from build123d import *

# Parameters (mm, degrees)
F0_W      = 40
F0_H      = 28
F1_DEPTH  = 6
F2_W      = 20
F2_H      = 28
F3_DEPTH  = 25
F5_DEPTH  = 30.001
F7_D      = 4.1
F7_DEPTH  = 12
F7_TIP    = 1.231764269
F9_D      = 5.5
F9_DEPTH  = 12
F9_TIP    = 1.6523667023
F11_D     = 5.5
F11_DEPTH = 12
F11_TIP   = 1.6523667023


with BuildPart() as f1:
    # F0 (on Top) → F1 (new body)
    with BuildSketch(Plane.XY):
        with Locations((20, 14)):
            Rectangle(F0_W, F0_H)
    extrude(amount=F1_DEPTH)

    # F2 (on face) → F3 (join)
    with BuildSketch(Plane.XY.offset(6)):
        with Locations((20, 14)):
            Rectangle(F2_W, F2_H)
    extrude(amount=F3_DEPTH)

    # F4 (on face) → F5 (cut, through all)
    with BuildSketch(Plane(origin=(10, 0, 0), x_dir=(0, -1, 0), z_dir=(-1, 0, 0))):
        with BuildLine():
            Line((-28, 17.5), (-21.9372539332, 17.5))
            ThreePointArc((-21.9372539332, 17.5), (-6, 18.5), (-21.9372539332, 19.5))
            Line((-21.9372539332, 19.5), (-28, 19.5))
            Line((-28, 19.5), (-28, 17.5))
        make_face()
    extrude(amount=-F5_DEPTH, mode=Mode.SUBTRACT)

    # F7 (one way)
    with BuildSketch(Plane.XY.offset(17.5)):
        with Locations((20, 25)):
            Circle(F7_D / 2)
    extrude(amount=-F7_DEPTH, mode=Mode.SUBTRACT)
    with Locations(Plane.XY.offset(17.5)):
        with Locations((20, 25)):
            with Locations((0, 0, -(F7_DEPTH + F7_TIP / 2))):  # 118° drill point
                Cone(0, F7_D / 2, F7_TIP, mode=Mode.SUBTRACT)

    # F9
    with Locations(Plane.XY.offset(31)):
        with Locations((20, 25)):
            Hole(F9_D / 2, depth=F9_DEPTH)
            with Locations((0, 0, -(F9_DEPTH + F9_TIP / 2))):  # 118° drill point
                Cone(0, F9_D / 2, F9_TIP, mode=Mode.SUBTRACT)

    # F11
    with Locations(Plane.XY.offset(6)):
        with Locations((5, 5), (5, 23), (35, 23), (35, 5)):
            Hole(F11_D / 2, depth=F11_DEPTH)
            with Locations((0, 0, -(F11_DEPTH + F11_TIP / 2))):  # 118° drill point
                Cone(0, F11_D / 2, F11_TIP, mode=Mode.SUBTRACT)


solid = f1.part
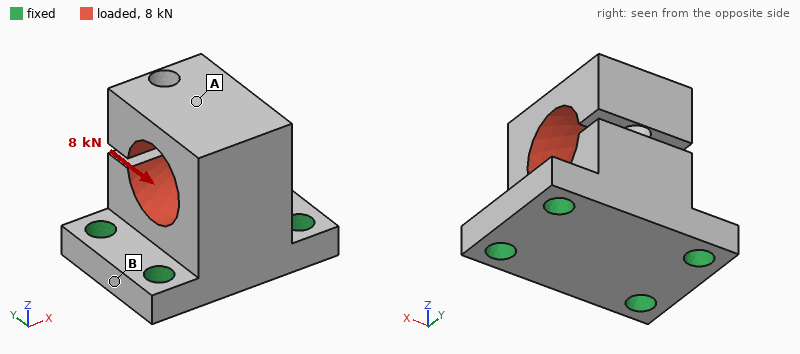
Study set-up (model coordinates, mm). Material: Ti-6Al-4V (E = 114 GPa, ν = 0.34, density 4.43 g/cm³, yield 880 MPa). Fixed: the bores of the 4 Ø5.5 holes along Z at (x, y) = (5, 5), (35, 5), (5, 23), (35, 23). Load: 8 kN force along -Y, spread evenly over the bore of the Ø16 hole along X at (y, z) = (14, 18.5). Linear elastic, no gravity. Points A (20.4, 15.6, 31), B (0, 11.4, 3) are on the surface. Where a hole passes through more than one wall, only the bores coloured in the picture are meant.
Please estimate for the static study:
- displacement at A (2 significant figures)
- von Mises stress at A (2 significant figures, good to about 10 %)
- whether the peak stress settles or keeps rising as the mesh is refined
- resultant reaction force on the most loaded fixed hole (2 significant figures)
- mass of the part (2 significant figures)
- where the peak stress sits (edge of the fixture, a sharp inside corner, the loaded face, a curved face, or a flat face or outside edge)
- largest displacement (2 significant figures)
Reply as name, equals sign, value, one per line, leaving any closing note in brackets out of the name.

displacement at A = 0.19 mm
von Mises stress at A = 79 MPa
whether the peak stress settles or keeps rising as the mesh is refined = keeps rising
resultant reaction force on the most loaded fixed hole = 4.2 kN
mass of the part = 68 g
where the peak stress sits = edge of the fixture
largest displacement = 0.22 mm
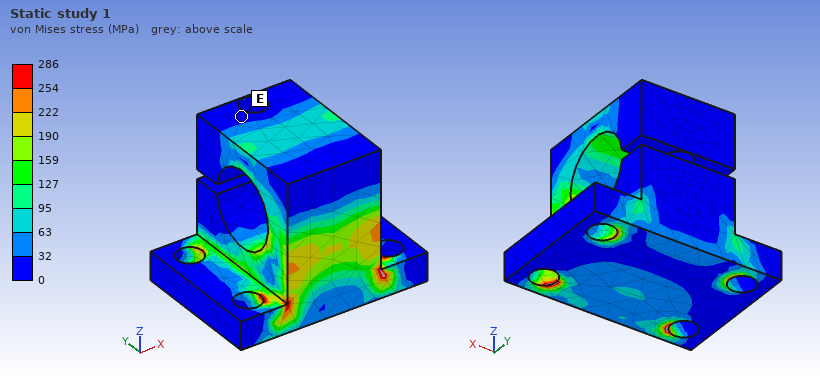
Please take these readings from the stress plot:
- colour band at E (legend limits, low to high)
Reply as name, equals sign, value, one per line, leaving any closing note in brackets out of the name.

colour band at E = 0 to 32 MPa
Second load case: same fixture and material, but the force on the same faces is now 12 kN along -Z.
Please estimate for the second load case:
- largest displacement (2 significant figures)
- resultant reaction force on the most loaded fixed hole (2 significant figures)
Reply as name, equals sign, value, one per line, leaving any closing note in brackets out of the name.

largest displacement = 0.66 mm
resultant reaction force on the most loaded fixed hole = 3.4 kN
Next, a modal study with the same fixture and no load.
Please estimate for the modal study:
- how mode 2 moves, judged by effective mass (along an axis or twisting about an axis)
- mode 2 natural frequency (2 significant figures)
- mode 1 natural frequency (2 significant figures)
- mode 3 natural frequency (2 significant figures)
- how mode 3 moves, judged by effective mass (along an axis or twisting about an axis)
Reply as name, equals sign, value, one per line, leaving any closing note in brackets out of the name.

how mode 2 moves, judged by effective mass = along X
mode 2 natural frequency = 5000 Hz
mode 1 natural frequency = 3600 Hz
mode 3 natural frequency = 7600 Hz
how mode 3 moves, judged by effective mass = along Y
